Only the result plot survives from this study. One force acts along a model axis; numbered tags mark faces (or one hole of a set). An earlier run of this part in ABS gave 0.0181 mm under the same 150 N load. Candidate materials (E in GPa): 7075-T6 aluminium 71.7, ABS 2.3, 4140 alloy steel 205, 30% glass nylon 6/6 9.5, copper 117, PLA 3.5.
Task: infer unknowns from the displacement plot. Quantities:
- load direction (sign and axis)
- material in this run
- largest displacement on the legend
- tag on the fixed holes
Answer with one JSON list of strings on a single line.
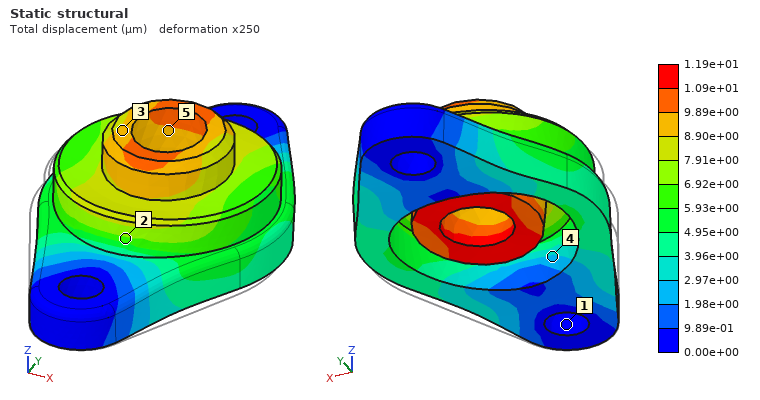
["+Y", "PLA", "1.19e+01 µm", "1"]
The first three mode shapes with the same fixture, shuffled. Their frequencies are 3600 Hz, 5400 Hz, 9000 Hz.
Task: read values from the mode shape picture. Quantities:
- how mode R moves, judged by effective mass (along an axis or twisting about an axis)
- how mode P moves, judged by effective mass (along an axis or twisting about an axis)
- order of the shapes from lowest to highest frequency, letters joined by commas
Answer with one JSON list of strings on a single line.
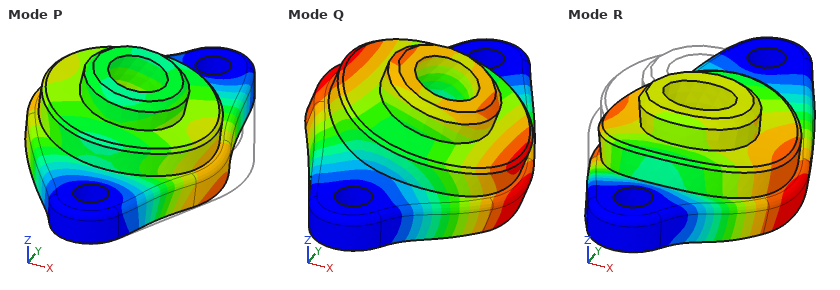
["along Z", "along X", "Q, R, P"]
